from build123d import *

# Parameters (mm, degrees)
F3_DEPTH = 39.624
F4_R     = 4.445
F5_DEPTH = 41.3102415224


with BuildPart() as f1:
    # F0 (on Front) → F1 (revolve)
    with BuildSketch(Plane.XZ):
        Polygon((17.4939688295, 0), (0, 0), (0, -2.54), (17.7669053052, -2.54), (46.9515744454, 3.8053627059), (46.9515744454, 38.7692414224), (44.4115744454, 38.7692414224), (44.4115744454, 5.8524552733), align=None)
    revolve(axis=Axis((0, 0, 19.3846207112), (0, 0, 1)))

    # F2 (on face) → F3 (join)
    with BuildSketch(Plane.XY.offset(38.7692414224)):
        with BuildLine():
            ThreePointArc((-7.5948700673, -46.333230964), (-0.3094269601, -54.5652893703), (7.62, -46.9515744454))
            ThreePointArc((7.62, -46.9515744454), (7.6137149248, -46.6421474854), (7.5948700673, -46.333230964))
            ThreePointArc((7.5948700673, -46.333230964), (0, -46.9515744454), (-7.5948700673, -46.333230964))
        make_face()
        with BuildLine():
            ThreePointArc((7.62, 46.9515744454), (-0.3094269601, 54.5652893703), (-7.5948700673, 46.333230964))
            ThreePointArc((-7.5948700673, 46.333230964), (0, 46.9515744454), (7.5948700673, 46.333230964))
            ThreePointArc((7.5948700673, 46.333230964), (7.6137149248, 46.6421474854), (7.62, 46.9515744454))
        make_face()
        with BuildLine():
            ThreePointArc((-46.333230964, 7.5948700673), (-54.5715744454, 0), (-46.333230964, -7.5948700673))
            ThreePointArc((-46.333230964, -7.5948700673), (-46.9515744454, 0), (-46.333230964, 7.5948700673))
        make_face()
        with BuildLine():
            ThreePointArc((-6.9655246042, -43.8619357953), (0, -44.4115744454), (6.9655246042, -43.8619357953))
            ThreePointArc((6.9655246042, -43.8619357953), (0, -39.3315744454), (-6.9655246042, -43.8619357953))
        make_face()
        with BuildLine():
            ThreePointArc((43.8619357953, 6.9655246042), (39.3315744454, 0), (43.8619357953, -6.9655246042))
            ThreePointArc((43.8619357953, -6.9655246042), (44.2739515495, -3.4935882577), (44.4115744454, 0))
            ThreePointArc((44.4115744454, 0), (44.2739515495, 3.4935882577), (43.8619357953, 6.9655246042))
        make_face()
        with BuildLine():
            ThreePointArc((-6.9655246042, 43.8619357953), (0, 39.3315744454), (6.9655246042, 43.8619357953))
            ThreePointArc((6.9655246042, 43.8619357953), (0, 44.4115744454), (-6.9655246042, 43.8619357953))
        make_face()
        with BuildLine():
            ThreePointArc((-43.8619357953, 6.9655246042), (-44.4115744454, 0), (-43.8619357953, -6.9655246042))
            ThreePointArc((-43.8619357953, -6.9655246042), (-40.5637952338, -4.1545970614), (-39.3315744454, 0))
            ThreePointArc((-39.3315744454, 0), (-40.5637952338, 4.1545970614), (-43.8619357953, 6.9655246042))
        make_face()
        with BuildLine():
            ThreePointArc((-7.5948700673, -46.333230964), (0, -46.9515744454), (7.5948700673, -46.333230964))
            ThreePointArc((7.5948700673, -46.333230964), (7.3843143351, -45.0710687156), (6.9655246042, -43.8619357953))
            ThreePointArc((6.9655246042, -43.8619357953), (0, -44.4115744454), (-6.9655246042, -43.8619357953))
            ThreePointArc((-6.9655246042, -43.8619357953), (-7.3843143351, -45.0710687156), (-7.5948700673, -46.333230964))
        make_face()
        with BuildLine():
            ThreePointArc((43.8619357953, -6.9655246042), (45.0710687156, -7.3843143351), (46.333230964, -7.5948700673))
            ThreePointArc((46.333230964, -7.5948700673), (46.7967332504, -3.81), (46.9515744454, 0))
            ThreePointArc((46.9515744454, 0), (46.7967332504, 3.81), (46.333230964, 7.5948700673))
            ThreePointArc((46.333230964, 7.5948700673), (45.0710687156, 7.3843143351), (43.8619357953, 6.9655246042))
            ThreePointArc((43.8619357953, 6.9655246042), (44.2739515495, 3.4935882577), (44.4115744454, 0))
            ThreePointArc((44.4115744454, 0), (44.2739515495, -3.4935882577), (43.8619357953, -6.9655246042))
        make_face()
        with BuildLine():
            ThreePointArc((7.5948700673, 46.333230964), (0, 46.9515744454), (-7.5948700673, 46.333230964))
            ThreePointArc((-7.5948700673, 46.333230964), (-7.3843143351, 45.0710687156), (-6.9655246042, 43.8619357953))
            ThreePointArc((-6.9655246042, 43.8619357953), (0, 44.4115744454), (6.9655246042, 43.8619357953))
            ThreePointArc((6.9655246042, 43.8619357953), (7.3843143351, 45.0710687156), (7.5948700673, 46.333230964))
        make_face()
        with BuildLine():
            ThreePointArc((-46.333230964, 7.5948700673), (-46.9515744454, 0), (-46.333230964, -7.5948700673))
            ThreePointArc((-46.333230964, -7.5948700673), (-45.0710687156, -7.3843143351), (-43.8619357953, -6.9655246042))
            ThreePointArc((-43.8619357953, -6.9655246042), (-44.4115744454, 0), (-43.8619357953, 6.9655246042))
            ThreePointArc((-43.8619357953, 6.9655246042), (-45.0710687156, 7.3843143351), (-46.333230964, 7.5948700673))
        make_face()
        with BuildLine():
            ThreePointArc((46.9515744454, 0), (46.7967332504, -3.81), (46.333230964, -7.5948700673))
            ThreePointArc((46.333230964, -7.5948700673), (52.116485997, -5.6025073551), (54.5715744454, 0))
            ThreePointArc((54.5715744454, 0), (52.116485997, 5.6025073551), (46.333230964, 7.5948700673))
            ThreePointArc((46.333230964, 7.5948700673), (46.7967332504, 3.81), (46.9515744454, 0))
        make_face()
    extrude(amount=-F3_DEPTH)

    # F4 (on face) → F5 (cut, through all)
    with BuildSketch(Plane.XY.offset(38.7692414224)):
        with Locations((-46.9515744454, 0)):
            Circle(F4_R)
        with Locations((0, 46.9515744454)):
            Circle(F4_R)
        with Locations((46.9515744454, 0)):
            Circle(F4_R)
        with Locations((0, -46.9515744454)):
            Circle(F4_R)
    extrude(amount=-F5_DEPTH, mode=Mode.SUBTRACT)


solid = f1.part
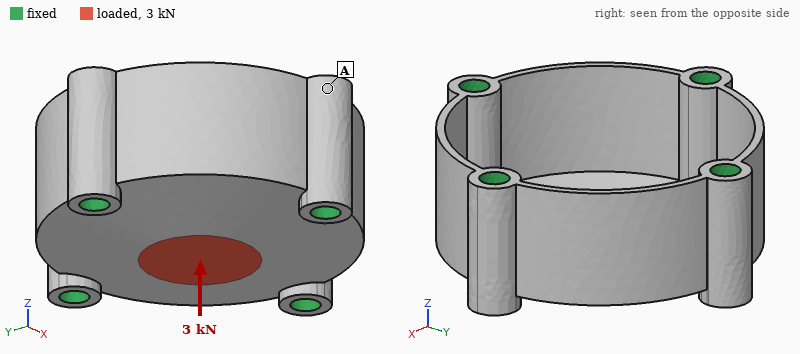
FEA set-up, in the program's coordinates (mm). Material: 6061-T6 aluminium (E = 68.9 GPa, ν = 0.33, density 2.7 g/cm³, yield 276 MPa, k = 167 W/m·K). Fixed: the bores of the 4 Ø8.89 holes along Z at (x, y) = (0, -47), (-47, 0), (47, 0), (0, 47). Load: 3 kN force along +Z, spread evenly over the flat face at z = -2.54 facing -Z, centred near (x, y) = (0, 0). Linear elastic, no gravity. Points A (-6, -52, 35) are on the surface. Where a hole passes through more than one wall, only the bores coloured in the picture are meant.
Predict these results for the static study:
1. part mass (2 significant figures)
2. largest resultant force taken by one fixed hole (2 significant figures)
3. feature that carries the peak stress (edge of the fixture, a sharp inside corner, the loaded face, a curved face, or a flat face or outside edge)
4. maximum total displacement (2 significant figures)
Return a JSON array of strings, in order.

["150 g", "2.5 kN", "the loaded face", "0.25 mm"]
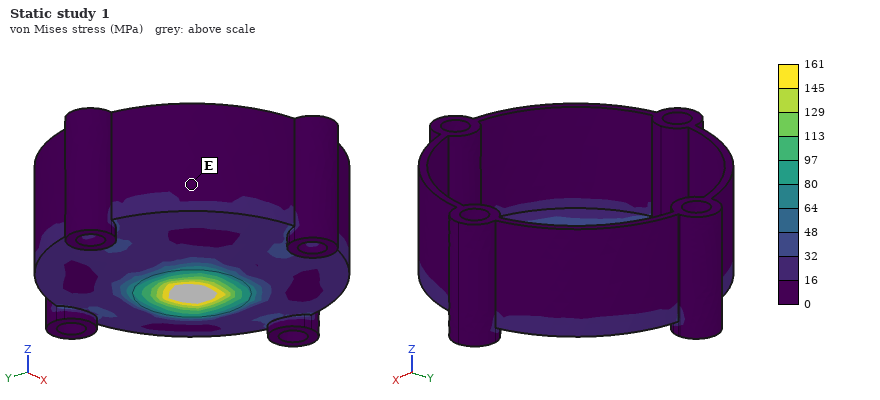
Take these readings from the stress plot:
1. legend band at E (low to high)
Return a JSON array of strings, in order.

["0 to 16 MPa"]
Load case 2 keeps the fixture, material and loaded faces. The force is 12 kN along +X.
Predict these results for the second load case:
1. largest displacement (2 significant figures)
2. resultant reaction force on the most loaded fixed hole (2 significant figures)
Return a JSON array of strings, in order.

["49 µm", "3.9 kN"]
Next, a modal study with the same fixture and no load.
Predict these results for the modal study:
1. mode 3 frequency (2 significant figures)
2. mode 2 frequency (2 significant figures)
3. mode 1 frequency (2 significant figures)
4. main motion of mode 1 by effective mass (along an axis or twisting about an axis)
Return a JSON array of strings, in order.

["8300 Hz", "8300 Hz", "6500 Hz", "along Z"]
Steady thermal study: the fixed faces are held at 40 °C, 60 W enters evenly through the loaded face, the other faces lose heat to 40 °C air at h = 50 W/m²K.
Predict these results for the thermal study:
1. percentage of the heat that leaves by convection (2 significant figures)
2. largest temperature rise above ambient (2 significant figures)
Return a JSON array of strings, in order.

["14 %", "34 K"]
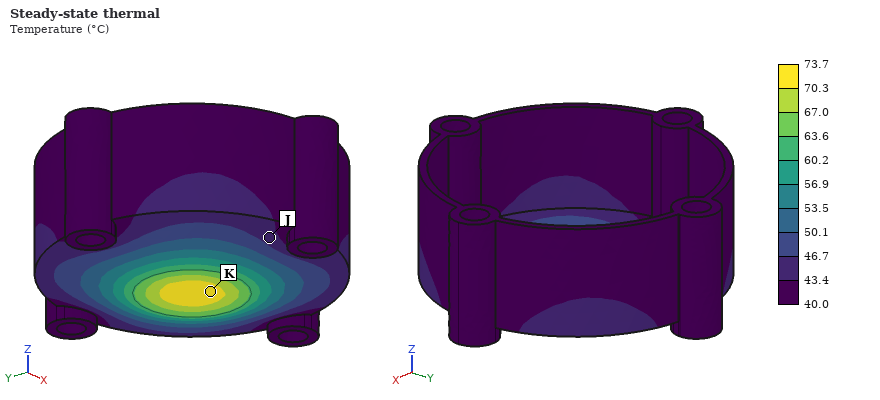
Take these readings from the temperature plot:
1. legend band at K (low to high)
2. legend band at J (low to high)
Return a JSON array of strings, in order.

["70.3 to 73.7 °C", "43.4 to 46.7 °C"]
